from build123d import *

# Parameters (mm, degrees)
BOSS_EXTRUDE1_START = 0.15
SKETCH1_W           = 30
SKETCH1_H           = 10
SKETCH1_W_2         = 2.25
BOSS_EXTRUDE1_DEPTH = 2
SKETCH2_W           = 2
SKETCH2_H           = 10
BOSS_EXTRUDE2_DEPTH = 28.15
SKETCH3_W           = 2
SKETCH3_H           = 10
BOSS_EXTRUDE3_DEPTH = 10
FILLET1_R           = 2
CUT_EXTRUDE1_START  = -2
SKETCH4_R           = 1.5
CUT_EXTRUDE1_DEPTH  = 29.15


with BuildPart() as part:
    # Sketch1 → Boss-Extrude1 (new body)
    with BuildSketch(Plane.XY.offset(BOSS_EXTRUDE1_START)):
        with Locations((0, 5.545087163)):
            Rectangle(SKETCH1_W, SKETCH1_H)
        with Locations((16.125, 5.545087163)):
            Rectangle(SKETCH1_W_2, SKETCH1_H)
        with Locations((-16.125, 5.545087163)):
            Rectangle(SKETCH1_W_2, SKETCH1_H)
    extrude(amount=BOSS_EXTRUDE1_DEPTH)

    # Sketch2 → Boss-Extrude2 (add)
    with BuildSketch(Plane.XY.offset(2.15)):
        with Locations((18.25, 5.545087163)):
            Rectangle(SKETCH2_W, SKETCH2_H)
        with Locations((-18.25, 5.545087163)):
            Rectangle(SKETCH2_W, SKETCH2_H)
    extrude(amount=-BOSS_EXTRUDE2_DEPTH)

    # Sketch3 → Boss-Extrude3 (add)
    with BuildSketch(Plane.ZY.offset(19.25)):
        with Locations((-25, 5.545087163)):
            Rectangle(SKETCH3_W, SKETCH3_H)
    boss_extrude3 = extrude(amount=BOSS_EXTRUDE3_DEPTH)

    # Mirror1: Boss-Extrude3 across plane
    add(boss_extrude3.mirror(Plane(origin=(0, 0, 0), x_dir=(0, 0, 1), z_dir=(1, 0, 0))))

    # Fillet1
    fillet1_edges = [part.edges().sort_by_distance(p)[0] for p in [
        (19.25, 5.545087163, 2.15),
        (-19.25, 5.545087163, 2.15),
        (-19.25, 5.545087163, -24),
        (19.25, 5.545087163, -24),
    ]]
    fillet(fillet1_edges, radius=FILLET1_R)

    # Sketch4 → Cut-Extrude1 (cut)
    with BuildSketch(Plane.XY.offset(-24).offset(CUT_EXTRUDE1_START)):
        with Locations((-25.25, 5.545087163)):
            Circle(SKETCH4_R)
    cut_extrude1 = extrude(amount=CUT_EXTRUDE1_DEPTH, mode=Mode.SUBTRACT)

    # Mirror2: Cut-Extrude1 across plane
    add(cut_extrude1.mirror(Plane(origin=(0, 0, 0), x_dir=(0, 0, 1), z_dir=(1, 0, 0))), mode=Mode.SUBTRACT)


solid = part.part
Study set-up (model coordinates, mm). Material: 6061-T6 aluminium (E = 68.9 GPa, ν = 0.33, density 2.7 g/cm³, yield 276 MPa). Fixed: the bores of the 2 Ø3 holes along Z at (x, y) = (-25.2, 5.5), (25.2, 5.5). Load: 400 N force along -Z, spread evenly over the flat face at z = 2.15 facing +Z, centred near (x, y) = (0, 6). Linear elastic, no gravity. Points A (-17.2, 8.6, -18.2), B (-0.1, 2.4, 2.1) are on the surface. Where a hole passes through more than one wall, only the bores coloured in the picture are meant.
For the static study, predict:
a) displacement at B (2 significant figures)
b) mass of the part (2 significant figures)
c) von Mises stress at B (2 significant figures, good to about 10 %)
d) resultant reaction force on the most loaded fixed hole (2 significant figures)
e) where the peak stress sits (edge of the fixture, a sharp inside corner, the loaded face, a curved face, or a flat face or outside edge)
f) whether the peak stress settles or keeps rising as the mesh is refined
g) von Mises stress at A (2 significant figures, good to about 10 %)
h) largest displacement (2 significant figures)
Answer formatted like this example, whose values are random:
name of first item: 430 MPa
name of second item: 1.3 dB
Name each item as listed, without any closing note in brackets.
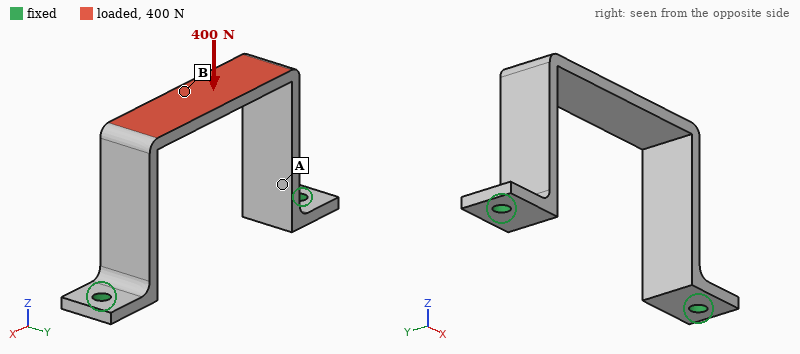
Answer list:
displacement at B: 0.23 mm
mass of the part: 5.9 g
von Mises stress at B: 140 MPa
resultant reaction force on the most loaded fixed hole: 210 N
where the peak stress sits: edge of the fixture
whether the peak stress settles or keeps rising as the mesh is refined: keeps rising
von Mises stress at A: 23 MPa
largest displacement: 0.24 mm
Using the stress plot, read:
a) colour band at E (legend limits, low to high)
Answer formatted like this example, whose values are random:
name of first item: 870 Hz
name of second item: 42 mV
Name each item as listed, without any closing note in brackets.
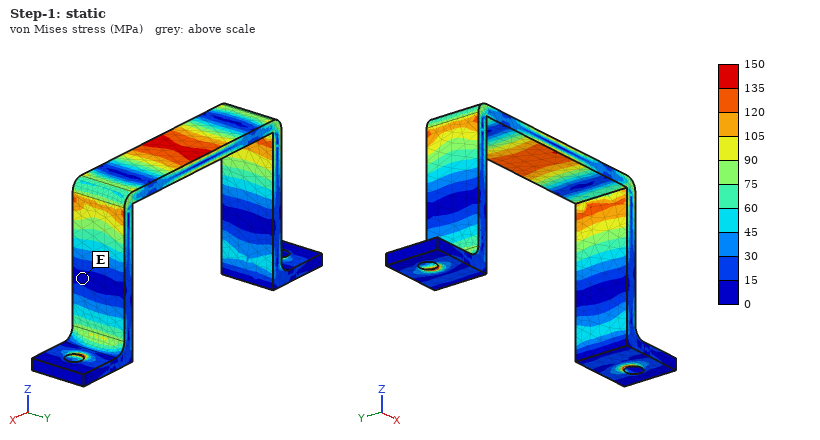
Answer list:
colour band at E: 0 to 15 MPa
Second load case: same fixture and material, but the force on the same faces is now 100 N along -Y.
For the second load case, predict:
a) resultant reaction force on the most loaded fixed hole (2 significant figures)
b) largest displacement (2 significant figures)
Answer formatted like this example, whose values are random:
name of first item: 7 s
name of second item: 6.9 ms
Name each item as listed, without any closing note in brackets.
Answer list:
resultant reaction force on the most loaded fixed hole: 50 N
largest displacement: 0.26 mm
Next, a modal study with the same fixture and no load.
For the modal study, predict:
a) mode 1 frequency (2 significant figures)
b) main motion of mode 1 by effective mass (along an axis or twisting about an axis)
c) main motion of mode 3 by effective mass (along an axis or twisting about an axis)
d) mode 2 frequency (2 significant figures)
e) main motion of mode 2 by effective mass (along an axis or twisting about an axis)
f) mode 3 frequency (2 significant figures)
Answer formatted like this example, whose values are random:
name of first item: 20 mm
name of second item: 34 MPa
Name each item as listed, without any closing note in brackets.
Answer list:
mode 1 frequency: 1700 Hz
main motion of mode 1 by effective mass: along X
main motion of mode 3 by effective mass: twisting about Z
mode 2 frequency: 1900 Hz
main motion of mode 2 by effective mass: along Y
mode 3 frequency: 3200 Hz
